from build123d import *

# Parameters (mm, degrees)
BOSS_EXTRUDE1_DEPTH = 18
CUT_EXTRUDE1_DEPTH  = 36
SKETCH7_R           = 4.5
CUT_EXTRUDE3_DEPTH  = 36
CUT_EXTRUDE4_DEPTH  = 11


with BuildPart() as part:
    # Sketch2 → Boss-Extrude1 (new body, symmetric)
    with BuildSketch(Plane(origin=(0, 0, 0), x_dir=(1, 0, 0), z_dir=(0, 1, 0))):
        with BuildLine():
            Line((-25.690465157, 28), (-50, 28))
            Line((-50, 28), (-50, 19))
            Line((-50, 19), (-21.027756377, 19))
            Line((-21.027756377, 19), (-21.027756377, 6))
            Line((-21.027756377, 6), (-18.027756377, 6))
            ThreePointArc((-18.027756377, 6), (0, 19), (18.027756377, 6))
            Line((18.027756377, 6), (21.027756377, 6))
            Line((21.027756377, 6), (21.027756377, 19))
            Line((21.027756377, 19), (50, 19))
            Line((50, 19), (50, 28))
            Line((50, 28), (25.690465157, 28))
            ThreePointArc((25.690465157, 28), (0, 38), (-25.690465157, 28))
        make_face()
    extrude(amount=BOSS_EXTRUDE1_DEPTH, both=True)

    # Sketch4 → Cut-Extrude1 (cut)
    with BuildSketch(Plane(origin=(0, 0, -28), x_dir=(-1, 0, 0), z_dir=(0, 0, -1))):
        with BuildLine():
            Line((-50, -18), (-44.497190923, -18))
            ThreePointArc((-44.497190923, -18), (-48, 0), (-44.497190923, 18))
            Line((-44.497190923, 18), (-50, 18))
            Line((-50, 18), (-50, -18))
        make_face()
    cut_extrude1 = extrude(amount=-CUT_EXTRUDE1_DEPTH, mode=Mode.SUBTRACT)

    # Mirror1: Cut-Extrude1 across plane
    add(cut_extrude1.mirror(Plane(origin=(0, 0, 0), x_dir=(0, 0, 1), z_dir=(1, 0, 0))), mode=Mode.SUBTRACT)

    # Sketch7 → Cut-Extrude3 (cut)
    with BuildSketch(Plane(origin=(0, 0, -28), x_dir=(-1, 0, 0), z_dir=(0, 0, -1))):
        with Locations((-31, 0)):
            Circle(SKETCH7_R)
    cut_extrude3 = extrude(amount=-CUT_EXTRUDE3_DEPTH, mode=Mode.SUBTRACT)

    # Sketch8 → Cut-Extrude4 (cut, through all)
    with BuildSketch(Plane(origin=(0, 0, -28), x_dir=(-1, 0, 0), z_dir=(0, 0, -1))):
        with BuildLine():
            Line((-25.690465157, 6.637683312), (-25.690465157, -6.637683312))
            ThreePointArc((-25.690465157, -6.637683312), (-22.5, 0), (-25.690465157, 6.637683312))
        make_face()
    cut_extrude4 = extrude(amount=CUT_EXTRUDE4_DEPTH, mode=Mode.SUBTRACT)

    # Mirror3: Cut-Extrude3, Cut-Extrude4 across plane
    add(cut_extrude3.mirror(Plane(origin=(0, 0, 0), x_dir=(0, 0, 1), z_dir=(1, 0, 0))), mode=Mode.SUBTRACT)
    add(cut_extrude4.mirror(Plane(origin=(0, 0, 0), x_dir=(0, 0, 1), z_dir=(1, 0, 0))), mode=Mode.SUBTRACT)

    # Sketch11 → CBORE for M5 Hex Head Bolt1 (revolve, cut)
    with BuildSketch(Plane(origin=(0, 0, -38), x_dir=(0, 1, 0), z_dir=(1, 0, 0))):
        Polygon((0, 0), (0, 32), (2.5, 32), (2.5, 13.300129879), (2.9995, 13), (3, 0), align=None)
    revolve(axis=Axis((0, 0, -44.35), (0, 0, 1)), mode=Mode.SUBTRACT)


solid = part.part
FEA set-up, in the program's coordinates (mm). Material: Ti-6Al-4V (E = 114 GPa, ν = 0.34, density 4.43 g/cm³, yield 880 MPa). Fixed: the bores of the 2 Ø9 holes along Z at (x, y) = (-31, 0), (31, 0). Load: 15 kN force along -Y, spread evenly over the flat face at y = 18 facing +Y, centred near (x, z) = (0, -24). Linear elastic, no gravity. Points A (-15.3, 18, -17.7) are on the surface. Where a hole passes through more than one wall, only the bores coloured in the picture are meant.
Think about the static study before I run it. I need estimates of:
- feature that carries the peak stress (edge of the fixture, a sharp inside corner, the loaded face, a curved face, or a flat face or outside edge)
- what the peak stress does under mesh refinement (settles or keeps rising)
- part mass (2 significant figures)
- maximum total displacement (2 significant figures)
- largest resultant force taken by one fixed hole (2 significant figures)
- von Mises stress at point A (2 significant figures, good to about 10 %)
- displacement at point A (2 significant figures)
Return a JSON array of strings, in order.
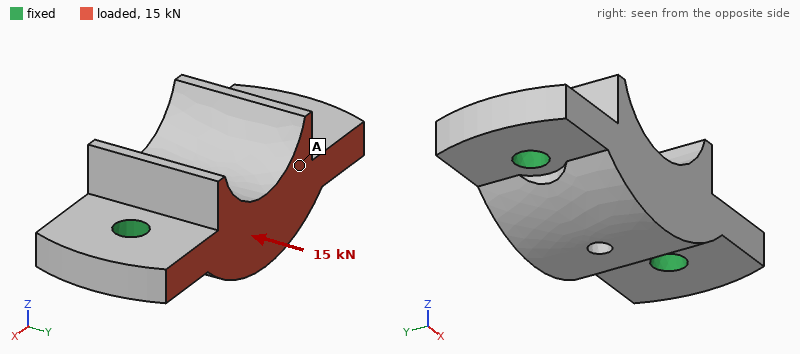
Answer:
["edge of the fixture", "keeps rising", "220 g", "15 µm", "7.5 kN", "17 MPa", "8.1 µm"]
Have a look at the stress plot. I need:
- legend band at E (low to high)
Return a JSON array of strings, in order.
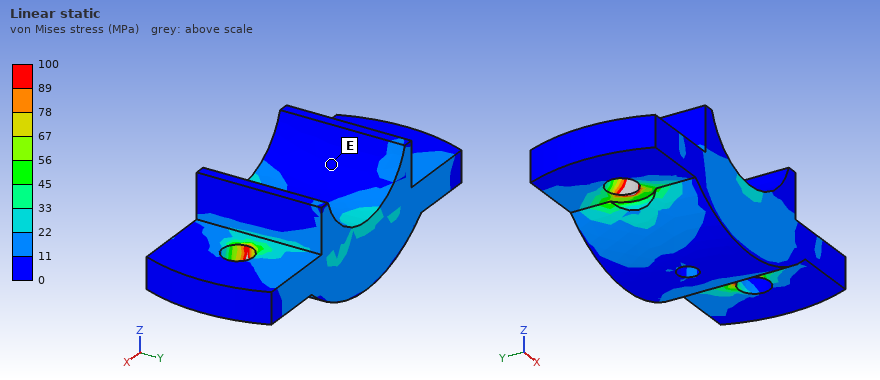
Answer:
["0 to 11 MPa"]
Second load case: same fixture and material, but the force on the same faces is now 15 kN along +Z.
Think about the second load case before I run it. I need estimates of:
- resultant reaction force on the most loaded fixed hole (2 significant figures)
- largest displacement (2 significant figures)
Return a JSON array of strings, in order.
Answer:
["7.8 kN", "84 µm"]
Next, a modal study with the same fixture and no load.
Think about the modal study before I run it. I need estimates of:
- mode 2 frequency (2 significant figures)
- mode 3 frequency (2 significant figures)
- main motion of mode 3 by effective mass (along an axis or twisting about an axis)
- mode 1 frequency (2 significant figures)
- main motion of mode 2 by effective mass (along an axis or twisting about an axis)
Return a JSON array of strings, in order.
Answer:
["12 kHz", "15 kHz", "along Y", "9000 Hz", "along Z"]
